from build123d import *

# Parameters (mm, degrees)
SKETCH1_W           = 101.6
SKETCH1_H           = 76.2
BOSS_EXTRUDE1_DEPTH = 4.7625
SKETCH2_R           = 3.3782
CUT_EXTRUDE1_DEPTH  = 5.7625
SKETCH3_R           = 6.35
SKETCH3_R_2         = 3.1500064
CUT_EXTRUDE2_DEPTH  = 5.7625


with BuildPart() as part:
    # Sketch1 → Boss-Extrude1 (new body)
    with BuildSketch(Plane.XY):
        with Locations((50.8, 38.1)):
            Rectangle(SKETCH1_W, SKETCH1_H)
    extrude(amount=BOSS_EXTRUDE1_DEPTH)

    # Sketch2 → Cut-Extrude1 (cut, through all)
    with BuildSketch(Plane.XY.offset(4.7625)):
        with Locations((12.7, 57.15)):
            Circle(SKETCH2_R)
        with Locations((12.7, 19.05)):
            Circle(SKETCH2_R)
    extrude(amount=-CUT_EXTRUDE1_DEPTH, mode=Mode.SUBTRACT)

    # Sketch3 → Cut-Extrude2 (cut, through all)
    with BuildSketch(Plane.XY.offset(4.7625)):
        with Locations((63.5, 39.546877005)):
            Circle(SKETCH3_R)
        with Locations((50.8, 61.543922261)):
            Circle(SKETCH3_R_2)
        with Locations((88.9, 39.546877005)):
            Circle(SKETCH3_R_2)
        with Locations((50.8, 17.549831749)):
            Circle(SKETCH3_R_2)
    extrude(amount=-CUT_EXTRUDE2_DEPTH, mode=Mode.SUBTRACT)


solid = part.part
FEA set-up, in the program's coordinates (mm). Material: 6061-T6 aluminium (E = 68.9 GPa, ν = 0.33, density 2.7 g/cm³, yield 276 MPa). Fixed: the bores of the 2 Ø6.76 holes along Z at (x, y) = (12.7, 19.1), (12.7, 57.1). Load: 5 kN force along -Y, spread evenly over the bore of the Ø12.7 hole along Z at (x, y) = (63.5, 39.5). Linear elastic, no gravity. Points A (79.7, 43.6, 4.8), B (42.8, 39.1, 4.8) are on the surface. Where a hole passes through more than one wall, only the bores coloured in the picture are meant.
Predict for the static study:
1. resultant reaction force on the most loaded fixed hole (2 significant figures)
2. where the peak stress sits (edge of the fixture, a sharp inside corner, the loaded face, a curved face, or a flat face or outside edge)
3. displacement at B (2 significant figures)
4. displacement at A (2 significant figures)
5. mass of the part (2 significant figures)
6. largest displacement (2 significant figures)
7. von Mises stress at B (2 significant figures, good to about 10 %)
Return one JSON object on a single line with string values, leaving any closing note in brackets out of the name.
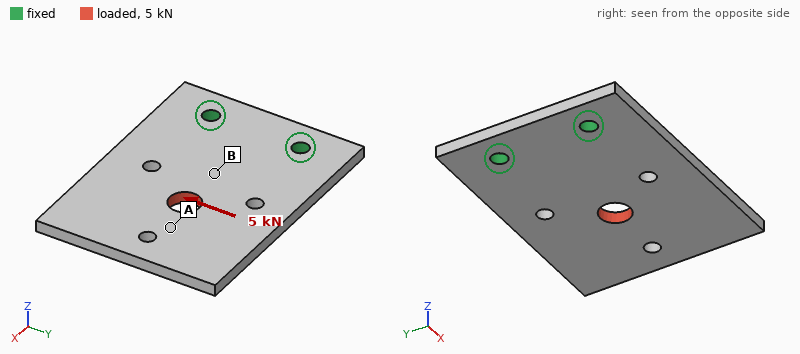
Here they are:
{"resultant reaction force on the most loaded fixed hole": "6.4 kN", "where the peak stress sits": "edge of the fixture", "displacement at B": "0.040 mm", "displacement at A": "0.094 mm", "mass of the part": "96 g", "largest displacement": "0.12 mm", "von Mises stress at B": "44 MPa"}
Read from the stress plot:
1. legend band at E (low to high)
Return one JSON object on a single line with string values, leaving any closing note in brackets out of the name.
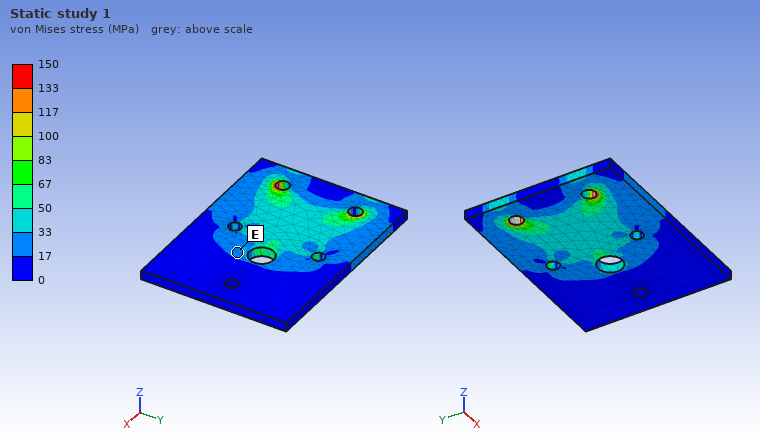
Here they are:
{"legend band at E": "17 to 33 MPa"}
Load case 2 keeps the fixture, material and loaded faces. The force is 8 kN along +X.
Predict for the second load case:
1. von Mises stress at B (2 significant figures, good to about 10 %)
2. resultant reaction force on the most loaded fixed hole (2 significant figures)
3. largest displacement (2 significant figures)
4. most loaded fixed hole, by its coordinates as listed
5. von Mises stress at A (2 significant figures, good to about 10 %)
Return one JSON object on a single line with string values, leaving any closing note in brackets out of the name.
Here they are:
{"von Mises stress at B": "35 MPa", "resultant reaction force on the most loaded fixed hole": "4.3 kN", "largest displacement": "33 µm", "most loaded fixed hole, by its coordinates as listed": "(12.7, 57.1)", "von Mises stress at A": "22 MPa"}
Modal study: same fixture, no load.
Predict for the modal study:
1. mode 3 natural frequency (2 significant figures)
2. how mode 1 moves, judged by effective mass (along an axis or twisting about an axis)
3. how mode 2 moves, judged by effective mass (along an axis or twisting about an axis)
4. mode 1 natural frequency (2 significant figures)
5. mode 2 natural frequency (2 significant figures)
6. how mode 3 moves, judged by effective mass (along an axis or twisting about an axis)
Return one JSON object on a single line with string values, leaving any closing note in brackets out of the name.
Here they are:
{"mode 3 natural frequency": "3000 Hz", "how mode 1 moves, judged by effective mass": "along Z", "how mode 2 moves, judged by effective mass": "twisting about X", "mode 1 natural frequency": "500 Hz", "mode 2 natural frequency": "1300 Hz", "how mode 3 moves, judged by effective mass": "along Z"}
